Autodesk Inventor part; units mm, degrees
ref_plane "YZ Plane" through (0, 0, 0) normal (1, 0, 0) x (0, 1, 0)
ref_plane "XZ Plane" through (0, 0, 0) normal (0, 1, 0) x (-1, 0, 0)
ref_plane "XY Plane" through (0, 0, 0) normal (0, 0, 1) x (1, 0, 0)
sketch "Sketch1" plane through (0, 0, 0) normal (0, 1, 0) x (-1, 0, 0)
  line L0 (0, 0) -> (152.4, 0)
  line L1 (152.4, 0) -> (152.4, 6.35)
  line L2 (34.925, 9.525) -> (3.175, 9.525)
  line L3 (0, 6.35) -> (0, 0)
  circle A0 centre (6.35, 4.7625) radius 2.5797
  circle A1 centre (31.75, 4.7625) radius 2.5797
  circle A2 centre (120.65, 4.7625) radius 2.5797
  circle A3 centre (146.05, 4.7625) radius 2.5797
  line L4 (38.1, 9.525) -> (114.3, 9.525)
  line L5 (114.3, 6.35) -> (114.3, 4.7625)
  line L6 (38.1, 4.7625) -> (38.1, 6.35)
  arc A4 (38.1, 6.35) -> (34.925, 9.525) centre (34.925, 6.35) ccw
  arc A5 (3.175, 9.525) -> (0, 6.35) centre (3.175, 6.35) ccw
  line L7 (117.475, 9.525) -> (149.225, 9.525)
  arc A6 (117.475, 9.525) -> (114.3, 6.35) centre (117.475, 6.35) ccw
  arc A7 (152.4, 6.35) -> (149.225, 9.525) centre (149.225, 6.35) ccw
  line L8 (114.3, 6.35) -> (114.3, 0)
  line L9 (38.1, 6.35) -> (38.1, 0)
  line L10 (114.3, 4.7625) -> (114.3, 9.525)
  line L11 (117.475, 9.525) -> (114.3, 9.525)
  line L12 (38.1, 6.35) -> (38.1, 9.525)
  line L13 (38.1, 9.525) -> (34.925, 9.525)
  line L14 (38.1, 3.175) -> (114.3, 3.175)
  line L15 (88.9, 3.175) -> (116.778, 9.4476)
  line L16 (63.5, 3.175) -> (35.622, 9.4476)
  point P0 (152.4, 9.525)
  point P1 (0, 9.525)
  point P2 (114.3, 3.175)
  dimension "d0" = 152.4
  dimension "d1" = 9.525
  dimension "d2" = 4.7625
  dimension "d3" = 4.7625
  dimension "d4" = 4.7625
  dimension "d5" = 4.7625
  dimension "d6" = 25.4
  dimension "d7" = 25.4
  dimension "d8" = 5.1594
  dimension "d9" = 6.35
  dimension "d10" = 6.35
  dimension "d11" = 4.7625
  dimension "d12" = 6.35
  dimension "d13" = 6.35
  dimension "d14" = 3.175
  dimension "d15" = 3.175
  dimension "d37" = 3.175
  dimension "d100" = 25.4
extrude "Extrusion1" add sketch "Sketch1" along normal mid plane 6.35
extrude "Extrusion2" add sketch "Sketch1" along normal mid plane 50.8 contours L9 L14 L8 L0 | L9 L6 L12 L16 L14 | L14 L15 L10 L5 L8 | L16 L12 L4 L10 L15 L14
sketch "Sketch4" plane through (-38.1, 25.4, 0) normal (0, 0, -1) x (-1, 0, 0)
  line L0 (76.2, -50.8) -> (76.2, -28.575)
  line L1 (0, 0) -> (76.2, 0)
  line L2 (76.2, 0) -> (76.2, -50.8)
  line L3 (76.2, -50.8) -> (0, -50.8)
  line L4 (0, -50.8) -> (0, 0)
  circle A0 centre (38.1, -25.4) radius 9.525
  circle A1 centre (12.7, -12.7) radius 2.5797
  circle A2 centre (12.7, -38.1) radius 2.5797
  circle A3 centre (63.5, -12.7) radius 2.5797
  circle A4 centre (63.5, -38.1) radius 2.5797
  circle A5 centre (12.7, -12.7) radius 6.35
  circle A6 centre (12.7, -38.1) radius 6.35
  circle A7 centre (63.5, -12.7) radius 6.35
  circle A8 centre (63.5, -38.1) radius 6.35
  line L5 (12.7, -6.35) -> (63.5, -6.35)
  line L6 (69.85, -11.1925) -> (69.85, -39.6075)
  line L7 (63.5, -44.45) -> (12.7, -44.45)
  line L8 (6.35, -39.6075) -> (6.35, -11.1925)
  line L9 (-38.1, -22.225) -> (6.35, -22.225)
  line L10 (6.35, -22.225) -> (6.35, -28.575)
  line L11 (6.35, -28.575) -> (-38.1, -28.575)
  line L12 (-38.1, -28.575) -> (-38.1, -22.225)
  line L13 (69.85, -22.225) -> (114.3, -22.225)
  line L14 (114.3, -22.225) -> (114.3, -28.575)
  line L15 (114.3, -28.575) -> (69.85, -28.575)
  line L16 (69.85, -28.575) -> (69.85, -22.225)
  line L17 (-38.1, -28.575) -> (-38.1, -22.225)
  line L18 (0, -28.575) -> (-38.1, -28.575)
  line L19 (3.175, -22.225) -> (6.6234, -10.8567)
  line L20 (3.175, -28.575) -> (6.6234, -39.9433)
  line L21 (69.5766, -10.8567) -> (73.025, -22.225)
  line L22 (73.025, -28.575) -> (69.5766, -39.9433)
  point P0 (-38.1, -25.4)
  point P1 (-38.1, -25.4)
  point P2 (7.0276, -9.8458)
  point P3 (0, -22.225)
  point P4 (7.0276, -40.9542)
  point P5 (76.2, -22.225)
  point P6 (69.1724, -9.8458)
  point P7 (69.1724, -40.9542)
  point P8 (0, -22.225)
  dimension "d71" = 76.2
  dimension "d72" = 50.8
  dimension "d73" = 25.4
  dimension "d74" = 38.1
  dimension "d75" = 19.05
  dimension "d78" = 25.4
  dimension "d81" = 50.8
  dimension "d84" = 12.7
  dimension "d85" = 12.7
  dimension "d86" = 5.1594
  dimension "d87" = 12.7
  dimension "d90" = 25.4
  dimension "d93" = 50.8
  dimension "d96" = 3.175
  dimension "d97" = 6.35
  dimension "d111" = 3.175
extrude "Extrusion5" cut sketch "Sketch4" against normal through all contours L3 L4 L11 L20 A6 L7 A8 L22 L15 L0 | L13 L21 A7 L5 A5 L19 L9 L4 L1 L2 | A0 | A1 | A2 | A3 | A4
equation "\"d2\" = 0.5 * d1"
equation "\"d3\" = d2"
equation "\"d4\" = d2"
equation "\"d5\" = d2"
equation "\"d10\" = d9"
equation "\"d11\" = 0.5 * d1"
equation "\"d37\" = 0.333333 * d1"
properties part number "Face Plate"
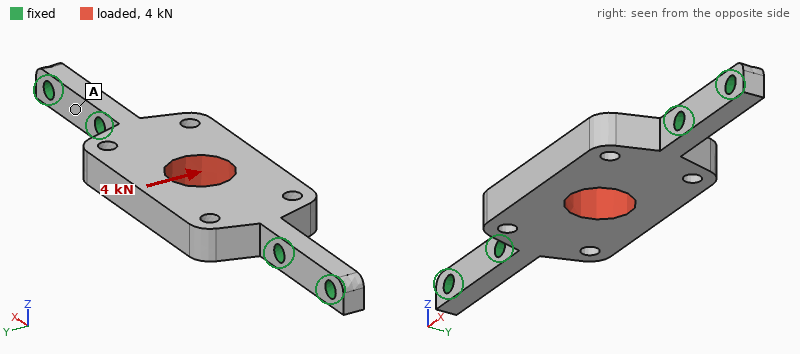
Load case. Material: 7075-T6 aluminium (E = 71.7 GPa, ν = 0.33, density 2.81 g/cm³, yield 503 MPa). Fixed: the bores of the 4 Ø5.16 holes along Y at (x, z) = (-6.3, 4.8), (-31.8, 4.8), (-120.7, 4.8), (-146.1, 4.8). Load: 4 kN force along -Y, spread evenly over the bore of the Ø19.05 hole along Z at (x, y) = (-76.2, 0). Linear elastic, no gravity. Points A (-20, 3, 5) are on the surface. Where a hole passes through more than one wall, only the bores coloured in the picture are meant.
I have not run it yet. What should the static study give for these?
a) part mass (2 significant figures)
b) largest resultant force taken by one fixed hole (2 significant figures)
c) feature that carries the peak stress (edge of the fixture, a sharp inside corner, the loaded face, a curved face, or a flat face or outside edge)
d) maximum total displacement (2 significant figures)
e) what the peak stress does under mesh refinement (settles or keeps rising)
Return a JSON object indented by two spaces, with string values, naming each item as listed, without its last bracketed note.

{
  "part mass": "69 g",
  "largest resultant force taken by one fixed hole": "2.0 kN",
  "feature that carries the peak stress": "edge of the fixture",
  "maximum total displacement": "44 µm",
  "what the peak stress does under mesh refinement": "keeps rising"
}
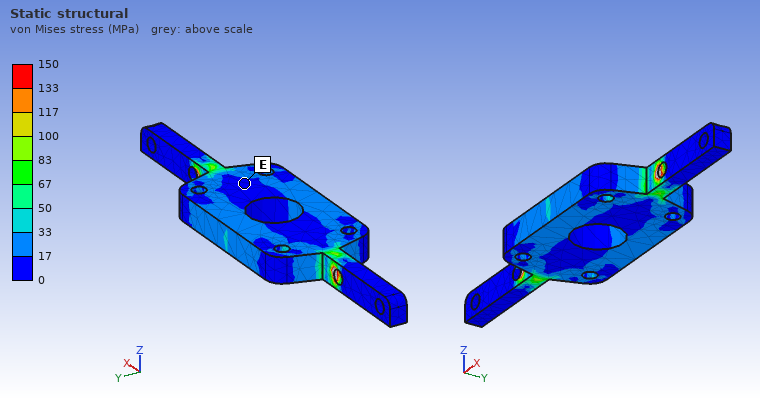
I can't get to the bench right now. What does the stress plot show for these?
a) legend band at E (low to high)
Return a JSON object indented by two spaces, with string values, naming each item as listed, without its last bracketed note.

{
  "legend band at E": "0 to 17 MPa"
}
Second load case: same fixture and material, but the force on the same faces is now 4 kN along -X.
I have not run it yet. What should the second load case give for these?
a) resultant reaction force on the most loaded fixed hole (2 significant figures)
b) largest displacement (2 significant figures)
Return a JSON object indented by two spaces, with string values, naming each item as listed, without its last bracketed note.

{
  "resultant reaction force on the most loaded fixed hole": "2.0 kN",
  "largest displacement": "9.5 µm"
}
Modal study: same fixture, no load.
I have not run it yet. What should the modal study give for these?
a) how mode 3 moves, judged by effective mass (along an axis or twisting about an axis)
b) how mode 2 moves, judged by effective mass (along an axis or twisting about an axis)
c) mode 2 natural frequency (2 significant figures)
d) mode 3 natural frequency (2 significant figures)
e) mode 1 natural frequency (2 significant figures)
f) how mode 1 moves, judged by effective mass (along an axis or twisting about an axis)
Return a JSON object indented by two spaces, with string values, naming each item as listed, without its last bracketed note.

{
  "how mode 3 moves, judged by effective mass": "along Y",
  "how mode 2 moves, judged by effective mass": "along Z",
  "mode 2 natural frequency": "3700 Hz",
  "mode 3 natural frequency": "7300 Hz",
  "mode 1 natural frequency": "3000 Hz",
  "how mode 1 moves, judged by effective mass": "twisting about X"
}
